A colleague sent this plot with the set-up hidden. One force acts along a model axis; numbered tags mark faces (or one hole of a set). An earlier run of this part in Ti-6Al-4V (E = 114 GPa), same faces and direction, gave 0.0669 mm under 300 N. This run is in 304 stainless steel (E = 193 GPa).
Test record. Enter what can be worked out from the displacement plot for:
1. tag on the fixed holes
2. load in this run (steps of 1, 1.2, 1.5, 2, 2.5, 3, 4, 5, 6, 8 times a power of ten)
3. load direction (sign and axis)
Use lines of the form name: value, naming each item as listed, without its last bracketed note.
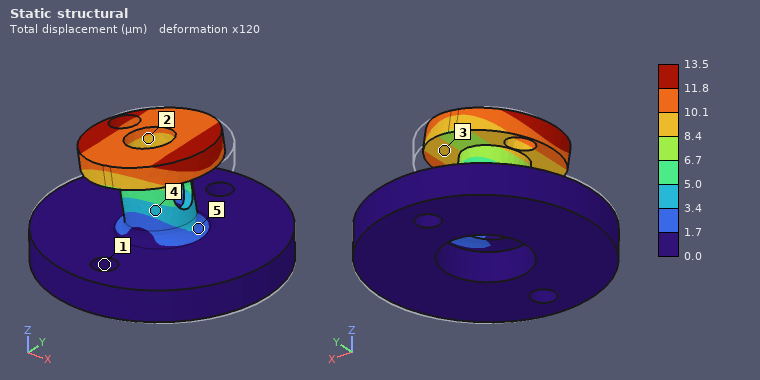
tag on the fixed holes: 1
load in this run: 100 N
load direction: -X
